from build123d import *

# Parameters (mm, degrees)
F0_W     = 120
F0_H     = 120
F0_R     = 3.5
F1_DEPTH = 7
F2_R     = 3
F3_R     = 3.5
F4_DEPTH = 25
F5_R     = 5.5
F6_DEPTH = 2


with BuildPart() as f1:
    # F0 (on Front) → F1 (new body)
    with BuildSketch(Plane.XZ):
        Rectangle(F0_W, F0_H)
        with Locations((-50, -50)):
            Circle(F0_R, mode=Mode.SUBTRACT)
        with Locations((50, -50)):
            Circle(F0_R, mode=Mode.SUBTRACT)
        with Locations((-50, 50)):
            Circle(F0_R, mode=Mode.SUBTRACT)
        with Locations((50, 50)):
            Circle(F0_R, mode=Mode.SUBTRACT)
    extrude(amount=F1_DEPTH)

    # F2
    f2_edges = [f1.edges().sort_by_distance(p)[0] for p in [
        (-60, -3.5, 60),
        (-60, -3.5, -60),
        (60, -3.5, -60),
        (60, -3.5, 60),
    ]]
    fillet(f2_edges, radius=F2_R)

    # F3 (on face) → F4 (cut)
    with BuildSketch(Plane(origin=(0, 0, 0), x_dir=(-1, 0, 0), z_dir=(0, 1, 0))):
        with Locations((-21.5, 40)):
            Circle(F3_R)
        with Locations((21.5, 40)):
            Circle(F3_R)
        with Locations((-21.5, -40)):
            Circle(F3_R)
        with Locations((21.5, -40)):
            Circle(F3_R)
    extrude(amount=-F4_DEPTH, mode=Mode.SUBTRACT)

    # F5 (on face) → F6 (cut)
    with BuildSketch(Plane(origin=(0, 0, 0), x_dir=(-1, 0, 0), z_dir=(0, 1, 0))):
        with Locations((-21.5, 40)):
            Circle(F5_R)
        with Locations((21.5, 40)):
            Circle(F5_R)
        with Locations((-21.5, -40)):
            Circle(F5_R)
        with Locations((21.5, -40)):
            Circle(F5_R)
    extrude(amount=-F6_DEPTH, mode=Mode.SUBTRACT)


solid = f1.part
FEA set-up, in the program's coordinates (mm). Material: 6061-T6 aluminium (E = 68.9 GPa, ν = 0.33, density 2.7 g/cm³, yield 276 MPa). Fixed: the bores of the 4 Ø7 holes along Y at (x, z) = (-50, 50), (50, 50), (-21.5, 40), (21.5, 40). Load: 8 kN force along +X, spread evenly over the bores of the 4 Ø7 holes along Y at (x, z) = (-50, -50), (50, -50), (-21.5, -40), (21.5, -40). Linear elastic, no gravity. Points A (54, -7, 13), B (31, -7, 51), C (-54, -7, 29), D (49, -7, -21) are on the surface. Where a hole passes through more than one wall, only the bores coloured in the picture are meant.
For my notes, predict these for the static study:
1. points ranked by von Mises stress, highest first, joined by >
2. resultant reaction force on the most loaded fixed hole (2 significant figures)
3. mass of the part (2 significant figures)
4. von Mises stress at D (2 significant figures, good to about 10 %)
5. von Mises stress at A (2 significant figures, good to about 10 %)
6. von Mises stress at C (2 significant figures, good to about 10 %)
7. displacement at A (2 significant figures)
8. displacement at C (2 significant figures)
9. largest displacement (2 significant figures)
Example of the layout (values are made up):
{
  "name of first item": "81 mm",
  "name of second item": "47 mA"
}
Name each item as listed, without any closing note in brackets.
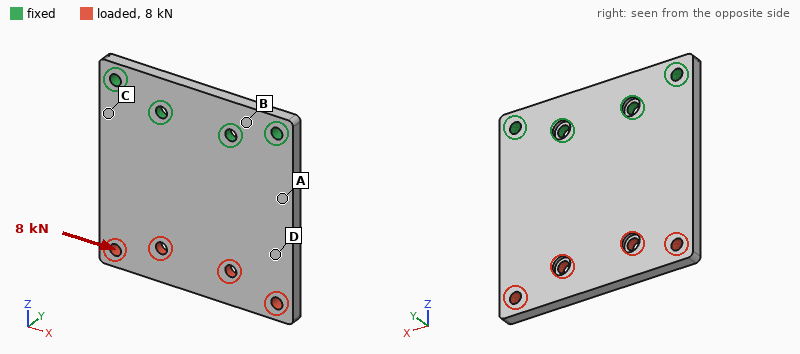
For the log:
{
  "points ranked by von Mises stress, highest first, joined by >": "C > A > D > B",
  "resultant reaction force on the most loaded fixed hole": "5.9 kN",
  "mass of the part": "260 g",
  "von Mises stress at D": "14 MPa",
  "von Mises stress at A": "26 MPa",
  "von Mises stress at C": "33 MPa",
  "displacement at A": "0.030 mm",
  "displacement at C": "0.016 mm",
  "largest displacement": "0.10 mm"
}
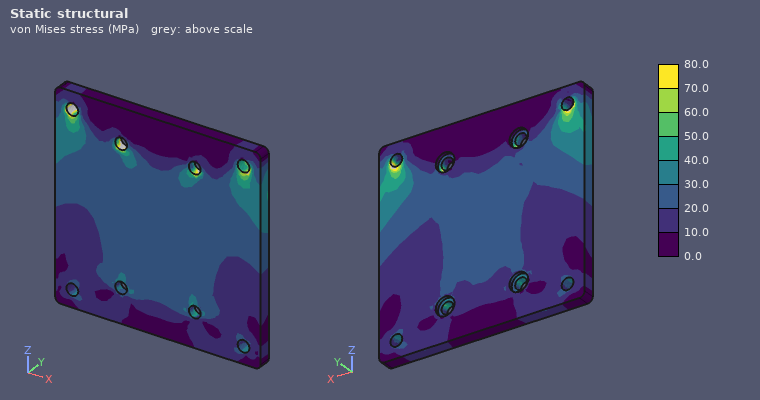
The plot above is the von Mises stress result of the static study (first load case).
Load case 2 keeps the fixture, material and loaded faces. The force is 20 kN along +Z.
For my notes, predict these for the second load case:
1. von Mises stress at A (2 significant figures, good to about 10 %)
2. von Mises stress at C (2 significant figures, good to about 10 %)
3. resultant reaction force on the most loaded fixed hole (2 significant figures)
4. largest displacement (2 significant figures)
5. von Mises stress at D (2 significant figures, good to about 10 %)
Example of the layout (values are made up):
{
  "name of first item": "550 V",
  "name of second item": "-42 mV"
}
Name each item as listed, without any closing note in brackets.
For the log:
{
  "von Mises stress at A": "32 MPa",
  "von Mises stress at C": "30 MPa",
  "resultant reaction force on the most loaded fixed hole": "5.8 kN",
  "largest displacement": "0.14 mm",
  "von Mises stress at D": "36 MPa"
}
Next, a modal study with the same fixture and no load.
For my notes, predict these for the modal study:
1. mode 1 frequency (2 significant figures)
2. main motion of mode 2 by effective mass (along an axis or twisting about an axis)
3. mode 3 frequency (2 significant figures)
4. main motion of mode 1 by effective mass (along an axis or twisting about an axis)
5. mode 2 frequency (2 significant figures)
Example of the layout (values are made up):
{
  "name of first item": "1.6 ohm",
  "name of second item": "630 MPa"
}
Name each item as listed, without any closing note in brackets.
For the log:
{
  "mode 1 frequency": "540 Hz",
  "main motion of mode 2 by effective mass": "twisting about Z",
  "mode 3 frequency": "2900 Hz",
  "main motion of mode 1 by effective mass": "along Y",
  "mode 2 frequency": "1100 Hz"
}
